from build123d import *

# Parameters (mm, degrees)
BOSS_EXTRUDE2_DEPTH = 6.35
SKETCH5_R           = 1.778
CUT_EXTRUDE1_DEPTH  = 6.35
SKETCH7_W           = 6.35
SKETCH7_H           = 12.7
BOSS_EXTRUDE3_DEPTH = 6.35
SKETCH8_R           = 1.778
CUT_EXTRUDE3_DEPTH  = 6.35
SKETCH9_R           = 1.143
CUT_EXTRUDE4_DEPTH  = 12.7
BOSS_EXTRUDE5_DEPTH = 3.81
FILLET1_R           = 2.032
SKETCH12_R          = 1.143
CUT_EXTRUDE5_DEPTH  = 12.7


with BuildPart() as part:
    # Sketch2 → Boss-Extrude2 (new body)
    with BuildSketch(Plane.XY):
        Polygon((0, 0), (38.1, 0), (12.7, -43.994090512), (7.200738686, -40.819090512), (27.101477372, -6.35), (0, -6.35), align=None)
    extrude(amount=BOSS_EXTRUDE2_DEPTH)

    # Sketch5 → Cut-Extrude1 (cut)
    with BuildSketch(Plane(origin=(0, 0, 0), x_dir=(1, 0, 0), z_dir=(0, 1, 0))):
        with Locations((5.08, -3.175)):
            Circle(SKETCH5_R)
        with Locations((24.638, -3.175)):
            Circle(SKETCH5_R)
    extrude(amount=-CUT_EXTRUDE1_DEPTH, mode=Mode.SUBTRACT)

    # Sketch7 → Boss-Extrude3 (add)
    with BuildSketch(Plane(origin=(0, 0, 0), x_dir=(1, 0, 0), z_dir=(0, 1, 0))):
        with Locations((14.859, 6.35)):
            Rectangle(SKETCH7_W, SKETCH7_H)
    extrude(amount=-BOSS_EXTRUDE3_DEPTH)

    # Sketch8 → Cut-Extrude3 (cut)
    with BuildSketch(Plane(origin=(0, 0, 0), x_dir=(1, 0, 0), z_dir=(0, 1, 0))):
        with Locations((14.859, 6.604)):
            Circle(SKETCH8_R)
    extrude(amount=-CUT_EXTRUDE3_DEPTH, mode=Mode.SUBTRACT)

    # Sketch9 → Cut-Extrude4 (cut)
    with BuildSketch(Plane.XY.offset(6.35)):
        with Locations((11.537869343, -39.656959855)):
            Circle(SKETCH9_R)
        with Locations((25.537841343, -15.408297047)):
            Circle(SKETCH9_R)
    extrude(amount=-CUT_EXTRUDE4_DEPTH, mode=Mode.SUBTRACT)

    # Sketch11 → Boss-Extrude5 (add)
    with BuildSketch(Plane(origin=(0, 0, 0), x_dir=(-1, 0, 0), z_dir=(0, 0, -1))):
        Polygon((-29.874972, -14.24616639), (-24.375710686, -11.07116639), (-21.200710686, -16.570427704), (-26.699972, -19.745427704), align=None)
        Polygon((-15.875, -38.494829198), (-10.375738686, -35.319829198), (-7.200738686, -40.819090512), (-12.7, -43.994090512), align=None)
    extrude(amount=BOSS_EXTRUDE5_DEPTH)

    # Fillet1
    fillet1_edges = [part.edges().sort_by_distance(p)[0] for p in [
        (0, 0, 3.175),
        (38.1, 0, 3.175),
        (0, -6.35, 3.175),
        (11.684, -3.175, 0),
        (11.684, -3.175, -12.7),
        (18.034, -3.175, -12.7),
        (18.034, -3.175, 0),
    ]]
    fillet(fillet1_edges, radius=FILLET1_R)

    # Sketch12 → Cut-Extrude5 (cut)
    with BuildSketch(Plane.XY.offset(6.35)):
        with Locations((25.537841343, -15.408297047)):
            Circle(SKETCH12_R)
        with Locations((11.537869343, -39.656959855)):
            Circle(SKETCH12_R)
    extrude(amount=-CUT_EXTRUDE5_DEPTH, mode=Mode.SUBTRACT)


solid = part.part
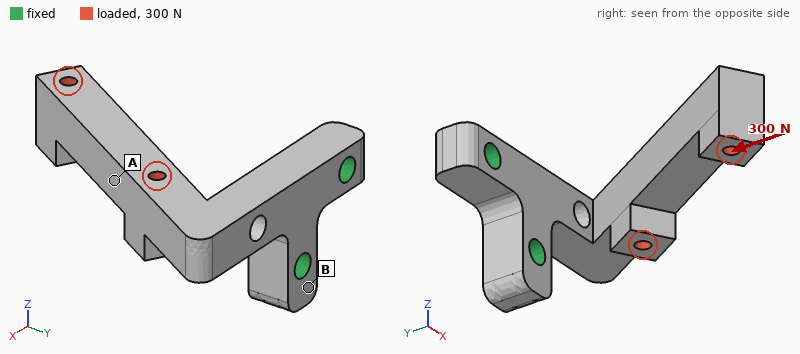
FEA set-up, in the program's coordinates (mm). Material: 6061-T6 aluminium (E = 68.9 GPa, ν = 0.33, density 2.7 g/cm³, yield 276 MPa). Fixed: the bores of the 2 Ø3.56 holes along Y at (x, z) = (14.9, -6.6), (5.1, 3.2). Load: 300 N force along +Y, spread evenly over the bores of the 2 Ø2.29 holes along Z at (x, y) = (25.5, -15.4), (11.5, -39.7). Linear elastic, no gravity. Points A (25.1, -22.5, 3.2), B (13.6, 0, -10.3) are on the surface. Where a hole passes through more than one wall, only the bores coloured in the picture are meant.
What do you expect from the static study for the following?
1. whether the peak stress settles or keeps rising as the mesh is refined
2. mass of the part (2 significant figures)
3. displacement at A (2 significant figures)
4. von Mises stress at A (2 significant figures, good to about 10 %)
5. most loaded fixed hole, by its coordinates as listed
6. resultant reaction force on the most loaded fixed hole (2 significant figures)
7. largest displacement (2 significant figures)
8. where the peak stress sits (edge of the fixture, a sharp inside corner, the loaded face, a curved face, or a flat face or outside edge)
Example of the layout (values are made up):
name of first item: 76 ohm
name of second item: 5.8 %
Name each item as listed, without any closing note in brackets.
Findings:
whether the peak stress settles or keeps rising as the mesh is refined: keeps rising
mass of the part: 9.9 g
displacement at A: 0.11 mm
von Mises stress at A: 35 MPa
most loaded fixed hole, by its coordinates as listed: (14.9, -6.6)
resultant reaction force on the most loaded fixed hole: 240 N
largest displacement: 0.33 mm
where the peak stress sits: a sharp inside corner
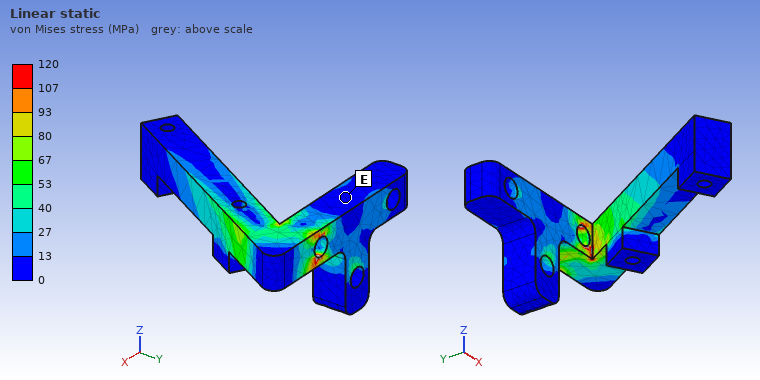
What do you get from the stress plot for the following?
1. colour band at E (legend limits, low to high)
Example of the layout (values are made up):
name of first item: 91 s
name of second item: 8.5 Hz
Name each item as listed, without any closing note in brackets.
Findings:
colour band at E: 0 to 13 MPa
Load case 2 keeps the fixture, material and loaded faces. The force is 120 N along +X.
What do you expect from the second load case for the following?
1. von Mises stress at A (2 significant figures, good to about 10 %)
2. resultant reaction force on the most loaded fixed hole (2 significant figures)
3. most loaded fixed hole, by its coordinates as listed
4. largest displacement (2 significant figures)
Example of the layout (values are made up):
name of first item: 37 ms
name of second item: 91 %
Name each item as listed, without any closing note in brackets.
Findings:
von Mises stress at A: 27 MPa
resultant reaction force on the most loaded fixed hole: 170 N
most loaded fixed hole, by its coordinates as listed: (5.1, 3.2)
largest displacement: 0.46 mm
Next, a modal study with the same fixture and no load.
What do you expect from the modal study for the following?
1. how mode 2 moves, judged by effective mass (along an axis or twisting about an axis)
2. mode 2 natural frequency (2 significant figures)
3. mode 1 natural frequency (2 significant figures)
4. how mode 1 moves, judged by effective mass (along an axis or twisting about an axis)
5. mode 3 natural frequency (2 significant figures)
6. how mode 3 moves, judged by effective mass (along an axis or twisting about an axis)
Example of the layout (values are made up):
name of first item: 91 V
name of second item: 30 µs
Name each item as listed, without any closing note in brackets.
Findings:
how mode 2 moves, judged by effective mass: along X
mode 2 natural frequency: 1500 Hz
mode 1 natural frequency: 1400 Hz
how mode 1 moves, judged by effective mass: along Z
mode 3 natural frequency: 5000 Hz
how mode 3 moves, judged by effective mass: along Y
